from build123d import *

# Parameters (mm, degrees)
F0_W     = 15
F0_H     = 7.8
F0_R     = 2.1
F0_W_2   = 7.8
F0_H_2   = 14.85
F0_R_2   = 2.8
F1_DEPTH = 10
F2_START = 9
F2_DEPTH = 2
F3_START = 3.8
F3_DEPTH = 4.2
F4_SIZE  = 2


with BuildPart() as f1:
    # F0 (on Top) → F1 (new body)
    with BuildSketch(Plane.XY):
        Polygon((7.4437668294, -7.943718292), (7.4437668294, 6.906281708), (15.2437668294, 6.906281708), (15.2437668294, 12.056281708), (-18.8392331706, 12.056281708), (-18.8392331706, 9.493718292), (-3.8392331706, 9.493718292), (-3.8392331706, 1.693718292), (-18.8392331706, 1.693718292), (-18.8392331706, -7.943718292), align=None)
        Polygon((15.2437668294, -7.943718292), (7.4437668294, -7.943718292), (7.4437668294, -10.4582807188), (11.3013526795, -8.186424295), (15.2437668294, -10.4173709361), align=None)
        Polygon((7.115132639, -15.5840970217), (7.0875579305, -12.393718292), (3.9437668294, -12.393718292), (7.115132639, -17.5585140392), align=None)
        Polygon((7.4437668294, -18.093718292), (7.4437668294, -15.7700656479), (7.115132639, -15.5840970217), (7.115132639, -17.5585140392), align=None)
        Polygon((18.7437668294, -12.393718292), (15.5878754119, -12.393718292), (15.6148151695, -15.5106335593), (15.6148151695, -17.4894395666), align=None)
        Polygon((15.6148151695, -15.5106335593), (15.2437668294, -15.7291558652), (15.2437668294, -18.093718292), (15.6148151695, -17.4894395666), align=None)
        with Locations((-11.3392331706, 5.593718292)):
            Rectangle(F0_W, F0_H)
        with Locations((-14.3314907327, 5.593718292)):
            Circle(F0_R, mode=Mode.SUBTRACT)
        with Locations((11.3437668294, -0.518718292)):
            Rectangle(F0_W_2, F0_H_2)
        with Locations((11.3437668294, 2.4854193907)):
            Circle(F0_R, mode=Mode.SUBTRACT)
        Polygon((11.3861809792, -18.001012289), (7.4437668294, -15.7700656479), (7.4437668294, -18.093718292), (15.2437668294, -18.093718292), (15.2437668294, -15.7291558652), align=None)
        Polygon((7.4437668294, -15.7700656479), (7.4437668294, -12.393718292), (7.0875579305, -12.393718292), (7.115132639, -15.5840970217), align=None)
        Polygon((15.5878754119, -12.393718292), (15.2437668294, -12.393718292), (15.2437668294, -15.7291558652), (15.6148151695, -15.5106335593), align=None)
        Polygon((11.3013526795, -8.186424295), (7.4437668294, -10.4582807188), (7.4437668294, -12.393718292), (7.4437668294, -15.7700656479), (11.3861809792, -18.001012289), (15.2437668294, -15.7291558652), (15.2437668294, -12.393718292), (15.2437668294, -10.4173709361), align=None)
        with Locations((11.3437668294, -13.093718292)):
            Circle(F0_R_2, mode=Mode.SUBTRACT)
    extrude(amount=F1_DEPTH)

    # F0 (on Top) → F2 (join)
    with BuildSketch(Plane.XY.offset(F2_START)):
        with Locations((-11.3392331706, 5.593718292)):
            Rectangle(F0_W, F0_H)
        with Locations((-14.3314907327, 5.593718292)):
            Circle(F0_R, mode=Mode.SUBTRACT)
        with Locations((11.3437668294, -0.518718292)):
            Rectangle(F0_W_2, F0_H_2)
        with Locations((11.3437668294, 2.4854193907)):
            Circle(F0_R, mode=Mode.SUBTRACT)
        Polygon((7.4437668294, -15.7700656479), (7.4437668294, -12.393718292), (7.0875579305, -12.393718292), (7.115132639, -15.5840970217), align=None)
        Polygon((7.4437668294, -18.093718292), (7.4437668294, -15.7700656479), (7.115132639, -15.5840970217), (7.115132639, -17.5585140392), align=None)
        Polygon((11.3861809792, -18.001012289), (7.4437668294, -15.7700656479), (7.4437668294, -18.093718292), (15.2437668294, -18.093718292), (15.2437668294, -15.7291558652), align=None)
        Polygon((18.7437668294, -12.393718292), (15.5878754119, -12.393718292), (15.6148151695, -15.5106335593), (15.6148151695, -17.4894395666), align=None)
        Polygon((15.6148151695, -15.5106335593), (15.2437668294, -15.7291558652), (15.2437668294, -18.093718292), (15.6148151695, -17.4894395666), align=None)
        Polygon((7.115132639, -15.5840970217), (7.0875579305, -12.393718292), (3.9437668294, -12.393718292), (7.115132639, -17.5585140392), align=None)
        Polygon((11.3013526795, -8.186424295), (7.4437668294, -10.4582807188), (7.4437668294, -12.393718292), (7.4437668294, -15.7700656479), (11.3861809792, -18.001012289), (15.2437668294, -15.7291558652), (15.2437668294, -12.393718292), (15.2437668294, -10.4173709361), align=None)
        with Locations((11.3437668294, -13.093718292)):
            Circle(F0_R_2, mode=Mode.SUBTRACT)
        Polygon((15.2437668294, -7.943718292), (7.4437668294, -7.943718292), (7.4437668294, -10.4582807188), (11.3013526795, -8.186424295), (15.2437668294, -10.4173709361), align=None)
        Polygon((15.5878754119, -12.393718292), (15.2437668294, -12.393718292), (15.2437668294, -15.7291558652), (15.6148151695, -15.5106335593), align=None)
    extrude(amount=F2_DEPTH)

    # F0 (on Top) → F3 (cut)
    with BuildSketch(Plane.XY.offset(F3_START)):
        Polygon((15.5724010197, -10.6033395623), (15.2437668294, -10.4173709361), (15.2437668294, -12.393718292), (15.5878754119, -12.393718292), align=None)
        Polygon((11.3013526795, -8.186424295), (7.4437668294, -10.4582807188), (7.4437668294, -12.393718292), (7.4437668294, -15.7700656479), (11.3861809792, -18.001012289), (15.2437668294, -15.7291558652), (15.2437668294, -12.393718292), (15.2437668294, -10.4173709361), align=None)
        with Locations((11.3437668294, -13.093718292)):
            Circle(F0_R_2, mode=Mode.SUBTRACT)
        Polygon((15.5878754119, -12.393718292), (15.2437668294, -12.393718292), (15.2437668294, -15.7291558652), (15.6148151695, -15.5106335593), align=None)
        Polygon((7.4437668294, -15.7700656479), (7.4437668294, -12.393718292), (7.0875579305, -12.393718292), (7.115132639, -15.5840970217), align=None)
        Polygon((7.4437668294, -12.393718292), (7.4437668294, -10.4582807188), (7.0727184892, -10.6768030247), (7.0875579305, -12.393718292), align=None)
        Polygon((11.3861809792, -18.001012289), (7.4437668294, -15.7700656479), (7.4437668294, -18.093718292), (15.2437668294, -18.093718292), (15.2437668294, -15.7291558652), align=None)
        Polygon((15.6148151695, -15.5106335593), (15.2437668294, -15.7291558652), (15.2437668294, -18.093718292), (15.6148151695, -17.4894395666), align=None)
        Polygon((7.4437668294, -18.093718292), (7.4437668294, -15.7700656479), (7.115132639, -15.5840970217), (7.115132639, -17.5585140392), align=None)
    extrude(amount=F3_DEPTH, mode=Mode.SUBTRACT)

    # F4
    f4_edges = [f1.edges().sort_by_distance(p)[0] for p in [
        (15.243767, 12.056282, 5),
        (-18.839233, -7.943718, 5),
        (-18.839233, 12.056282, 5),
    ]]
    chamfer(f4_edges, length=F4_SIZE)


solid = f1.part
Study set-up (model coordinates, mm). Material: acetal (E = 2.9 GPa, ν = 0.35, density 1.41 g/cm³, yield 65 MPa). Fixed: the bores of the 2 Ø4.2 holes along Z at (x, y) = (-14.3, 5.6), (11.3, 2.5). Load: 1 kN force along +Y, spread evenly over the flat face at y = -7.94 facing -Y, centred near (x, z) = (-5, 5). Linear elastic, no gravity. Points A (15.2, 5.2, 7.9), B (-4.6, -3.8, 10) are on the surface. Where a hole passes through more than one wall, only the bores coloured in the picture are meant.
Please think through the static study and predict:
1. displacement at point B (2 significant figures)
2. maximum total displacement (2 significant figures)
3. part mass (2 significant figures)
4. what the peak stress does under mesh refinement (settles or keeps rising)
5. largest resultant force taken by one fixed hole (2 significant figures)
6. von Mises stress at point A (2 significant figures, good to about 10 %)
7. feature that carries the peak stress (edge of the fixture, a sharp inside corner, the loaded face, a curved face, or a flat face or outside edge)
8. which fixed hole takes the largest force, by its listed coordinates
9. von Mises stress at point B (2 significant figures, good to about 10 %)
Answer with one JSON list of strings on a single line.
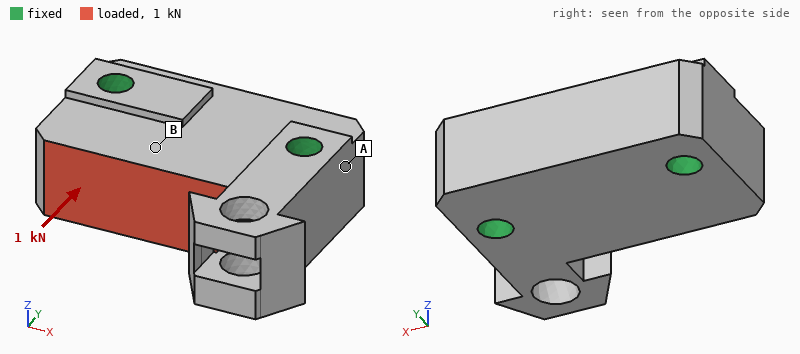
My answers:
["25 µm", "33 µm", "10 g", "keeps rising", "650 N", "1.2 MPa", "edge of the fixture", "(-14.3, 5.6)", "3.6 MPa"]
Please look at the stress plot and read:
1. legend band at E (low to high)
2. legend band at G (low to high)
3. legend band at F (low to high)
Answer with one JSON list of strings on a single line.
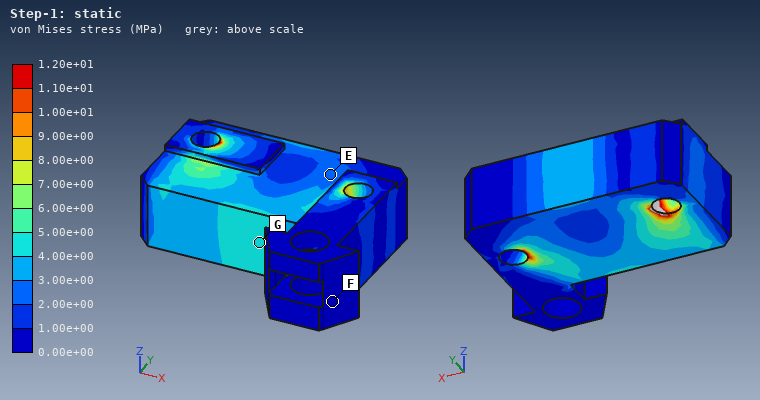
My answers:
["2.00e+00 to 3.00e+00 MPa", "4.00e+00 to 5.00e+00 MPa", "0.00e+00 to 1.00e+00 MPa"]
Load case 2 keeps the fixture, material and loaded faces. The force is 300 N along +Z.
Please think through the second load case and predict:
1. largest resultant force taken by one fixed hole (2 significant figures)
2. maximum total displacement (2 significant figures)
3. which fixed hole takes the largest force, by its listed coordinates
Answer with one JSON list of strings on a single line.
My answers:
["170 N", "62 µm", "(-14.3, 5.6)"]
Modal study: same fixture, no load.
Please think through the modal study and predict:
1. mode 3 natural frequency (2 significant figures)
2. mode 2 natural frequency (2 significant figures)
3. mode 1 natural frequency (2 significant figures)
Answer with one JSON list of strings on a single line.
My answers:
["8100 Hz", "5700 Hz", "5200 Hz"]
